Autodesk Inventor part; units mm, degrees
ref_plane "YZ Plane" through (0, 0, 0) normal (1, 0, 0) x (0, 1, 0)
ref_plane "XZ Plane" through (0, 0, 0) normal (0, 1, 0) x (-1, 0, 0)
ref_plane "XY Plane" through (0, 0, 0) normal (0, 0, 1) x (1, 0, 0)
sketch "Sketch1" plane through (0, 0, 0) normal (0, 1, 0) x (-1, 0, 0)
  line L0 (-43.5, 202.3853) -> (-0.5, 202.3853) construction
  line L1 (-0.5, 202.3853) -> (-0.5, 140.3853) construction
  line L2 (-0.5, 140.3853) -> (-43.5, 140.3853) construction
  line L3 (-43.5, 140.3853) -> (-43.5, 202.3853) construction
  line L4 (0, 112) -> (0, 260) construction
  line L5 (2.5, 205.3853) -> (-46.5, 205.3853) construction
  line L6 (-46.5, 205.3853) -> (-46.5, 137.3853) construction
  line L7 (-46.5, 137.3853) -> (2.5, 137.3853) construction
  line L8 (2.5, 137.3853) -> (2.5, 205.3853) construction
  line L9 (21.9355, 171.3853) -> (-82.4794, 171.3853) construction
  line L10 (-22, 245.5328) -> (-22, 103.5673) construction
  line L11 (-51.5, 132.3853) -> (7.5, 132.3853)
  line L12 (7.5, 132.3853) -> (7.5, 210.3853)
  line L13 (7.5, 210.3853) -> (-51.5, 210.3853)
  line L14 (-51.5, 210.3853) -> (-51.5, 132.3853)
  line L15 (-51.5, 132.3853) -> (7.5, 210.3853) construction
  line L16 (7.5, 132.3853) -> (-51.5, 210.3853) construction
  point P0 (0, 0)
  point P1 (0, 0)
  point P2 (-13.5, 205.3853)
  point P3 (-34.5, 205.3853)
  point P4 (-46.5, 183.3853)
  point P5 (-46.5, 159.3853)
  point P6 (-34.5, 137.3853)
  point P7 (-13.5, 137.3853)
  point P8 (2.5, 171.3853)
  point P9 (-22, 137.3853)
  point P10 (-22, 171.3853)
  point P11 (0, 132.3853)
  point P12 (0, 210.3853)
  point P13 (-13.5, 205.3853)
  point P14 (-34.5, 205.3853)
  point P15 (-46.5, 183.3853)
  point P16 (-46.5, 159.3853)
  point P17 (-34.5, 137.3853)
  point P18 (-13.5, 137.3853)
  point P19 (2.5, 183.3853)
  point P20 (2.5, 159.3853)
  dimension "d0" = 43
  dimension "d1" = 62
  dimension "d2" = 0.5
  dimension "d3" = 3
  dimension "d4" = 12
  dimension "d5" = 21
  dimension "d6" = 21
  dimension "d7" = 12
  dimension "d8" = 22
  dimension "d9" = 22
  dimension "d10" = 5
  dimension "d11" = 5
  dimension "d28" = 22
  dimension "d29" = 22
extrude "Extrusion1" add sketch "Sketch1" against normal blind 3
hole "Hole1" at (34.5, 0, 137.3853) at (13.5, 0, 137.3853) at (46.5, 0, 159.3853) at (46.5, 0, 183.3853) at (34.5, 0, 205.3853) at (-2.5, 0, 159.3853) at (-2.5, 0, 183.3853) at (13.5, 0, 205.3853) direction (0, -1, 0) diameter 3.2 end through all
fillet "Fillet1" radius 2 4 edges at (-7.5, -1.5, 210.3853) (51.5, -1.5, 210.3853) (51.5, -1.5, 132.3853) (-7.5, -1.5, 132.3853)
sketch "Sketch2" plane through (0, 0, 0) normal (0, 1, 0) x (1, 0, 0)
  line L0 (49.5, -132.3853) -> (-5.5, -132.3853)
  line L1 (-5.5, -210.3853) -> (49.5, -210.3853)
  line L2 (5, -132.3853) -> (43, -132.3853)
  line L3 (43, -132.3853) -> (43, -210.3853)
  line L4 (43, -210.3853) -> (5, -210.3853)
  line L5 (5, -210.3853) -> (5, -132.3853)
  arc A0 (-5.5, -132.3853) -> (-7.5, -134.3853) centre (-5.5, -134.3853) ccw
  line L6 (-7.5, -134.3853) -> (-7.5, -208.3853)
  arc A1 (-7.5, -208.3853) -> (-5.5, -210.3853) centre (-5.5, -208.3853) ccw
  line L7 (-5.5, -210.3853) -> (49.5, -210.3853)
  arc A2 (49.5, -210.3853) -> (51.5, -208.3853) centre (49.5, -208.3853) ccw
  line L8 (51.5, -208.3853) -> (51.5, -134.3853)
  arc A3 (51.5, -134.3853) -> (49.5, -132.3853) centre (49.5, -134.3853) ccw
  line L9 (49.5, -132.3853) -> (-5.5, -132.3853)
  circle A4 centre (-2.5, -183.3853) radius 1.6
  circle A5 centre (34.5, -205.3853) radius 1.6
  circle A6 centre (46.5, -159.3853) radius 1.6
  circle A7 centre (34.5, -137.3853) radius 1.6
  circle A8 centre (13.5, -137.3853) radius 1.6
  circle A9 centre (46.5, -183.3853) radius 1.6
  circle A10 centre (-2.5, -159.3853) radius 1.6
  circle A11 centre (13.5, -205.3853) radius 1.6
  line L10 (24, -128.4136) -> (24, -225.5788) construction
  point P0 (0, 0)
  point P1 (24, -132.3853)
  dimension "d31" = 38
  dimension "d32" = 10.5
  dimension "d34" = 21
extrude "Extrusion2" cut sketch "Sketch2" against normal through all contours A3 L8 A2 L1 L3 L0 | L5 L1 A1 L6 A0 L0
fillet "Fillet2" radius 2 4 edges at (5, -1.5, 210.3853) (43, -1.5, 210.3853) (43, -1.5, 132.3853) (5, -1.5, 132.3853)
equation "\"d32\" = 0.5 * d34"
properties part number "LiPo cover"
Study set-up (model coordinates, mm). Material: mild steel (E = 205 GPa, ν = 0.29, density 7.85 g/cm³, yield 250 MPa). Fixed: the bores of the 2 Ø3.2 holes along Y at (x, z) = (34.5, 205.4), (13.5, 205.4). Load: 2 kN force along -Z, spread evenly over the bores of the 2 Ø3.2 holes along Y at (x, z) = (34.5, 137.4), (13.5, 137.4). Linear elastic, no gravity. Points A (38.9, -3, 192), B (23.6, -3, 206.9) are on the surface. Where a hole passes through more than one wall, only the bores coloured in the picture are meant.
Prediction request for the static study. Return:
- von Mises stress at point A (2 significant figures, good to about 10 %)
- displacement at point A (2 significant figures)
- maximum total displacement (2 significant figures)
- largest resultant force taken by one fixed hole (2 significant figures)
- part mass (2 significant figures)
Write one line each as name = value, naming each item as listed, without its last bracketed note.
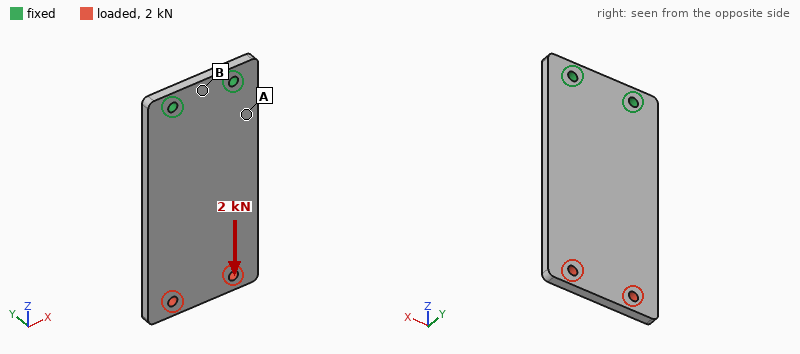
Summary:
von Mises stress at point A = 18 MPa
displacement at point A = 1.7 µm
maximum total displacement = 7.4 µm
largest resultant force taken by one fixed hole = 1.0 kN
part mass = 69 g
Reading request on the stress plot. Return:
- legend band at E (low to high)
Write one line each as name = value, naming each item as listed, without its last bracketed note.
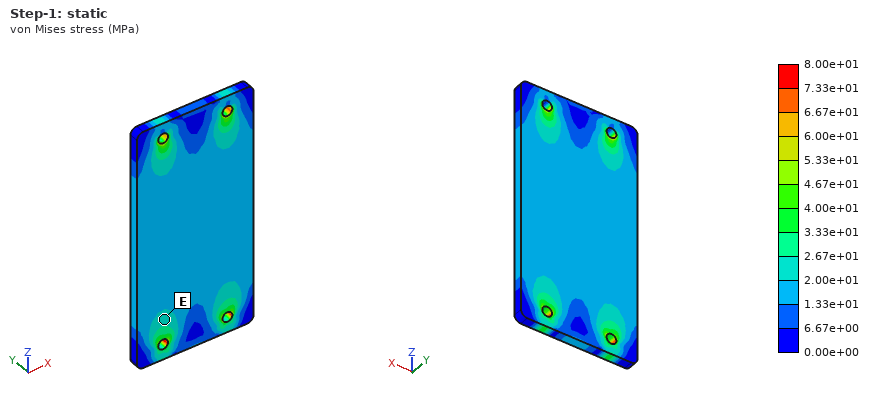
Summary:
legend band at E = 2.00e+01 to 2.67e+01 MPa
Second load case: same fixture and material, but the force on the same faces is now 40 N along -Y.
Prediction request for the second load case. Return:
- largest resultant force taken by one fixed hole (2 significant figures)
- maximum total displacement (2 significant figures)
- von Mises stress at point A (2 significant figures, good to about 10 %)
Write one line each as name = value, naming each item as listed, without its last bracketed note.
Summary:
largest resultant force taken by one fixed hole = 20 N
maximum total displacement = 0.27 mm
von Mises stress at point A = 38 MPa
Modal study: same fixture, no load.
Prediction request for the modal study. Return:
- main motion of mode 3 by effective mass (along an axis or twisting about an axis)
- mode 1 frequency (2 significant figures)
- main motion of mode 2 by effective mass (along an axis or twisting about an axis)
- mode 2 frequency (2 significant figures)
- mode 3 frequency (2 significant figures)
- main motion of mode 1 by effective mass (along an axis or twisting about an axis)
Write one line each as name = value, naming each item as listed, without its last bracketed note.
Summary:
main motion of mode 3 by effective mass = along Y
mode 1 frequency = 470 Hz
main motion of mode 2 by effective mass = twisting about Z
mode 2 frequency = 1900 Hz
mode 3 frequency = 2900 Hz
main motion of mode 1 by effective mass = along Y
